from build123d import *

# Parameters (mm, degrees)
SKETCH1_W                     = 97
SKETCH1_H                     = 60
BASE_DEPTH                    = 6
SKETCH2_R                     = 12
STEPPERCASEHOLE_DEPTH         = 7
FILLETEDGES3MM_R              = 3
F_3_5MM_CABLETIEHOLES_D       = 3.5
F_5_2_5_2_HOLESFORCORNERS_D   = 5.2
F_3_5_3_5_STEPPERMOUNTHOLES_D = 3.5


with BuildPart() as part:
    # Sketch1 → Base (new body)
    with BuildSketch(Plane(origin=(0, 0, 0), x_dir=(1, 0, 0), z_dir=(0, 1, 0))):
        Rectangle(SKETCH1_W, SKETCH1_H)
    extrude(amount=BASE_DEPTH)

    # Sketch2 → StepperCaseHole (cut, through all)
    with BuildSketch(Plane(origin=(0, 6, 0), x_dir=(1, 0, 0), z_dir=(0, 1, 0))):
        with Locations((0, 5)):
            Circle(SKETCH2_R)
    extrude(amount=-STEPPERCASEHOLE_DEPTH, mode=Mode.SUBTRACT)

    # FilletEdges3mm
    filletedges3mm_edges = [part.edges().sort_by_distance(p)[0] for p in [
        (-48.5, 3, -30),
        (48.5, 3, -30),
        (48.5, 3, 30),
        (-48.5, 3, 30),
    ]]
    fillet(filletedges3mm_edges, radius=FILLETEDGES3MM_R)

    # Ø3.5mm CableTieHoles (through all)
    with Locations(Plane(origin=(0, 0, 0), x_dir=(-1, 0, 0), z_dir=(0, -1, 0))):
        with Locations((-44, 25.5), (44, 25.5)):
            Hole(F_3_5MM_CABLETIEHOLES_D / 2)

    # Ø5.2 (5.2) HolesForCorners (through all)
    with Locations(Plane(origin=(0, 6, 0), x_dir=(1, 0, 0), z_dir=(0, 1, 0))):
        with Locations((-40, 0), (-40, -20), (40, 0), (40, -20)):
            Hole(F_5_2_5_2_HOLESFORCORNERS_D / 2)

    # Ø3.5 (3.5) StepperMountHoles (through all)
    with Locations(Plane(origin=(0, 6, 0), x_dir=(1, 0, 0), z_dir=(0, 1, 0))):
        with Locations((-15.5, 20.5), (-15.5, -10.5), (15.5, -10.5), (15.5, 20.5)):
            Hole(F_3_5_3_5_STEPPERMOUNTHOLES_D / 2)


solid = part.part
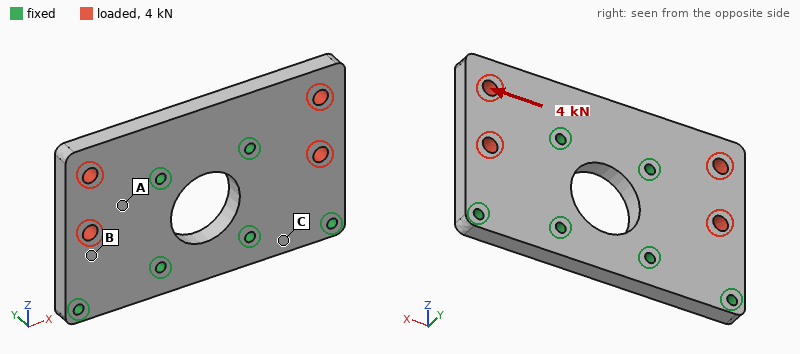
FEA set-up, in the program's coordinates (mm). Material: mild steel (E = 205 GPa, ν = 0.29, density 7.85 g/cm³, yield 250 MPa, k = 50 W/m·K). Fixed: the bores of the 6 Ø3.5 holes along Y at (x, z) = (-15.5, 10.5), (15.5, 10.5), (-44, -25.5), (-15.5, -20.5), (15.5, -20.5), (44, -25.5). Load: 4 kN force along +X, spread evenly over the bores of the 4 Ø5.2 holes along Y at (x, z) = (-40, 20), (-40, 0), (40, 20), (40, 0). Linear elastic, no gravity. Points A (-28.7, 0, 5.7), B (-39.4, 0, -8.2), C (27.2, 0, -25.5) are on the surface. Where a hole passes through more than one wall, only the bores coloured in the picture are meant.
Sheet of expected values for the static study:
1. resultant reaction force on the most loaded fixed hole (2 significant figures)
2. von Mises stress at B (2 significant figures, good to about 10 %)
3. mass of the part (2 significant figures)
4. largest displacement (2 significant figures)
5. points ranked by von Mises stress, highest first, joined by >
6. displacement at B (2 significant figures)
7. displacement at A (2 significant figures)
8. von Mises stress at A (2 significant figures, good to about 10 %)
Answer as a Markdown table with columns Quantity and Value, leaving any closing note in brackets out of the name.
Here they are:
| Quantity | Value |
|---|---|
| resultant reaction force on the most loaded fixed hole | 1.5 kN |
| von Mises stress at B | 5.1 MPa |
| mass of the part | 250 g |
| largest displacement | 2.2 µm |
| points ranked by von Mises stress, highest first, joined by > | A > B > C |
| displacement at B | 0.73 µm |
| displacement at A | 0.86 µm |
| von Mises stress at A | 9.9 MPa |
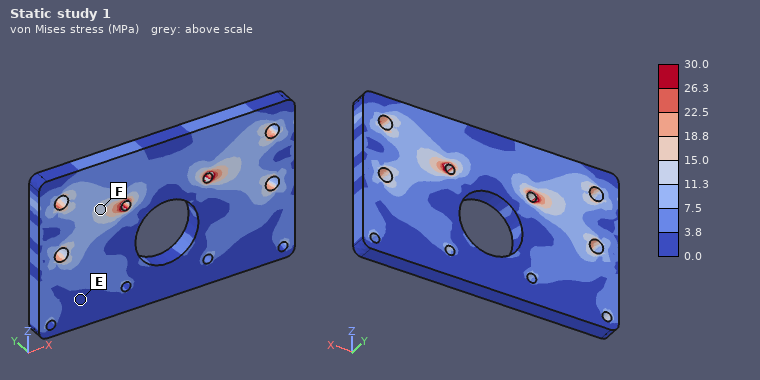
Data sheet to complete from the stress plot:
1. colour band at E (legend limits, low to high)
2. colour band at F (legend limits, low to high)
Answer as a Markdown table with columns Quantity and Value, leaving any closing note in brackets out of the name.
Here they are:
| Quantity | Value |
|---|---|
| colour band at E | 0.0 to 3.8 MPa |
| colour band at F | 11.3 to 15.0 MPa |
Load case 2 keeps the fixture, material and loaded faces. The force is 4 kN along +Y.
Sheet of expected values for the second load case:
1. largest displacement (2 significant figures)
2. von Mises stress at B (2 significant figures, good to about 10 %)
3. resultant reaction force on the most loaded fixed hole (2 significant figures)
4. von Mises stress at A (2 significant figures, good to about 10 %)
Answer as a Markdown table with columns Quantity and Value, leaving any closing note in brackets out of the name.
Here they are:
| Quantity | Value |
|---|---|
| largest displacement | 99 µm |
| von Mises stress at B | 76 MPa |
| resultant reaction force on the most loaded fixed hole | 1.5 kN |
| von Mises stress at A | 66 MPa |
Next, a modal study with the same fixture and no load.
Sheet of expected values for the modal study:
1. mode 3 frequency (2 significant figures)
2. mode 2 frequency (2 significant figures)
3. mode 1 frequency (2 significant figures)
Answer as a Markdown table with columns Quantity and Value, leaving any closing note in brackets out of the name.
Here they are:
| Quantity | Value |
|---|---|
| mode 3 frequency | 9700 Hz |
| mode 2 frequency | 5100 Hz |
| mode 1 frequency | 5000 Hz |
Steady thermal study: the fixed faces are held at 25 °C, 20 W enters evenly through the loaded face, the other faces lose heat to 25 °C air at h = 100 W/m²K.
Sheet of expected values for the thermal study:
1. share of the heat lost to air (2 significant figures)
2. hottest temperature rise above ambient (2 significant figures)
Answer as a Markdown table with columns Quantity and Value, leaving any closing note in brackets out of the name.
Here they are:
| Quantity | Value |
|---|---|
| share of the heat lost to air | 33 % |
| hottest temperature rise above ambient | 17 K |
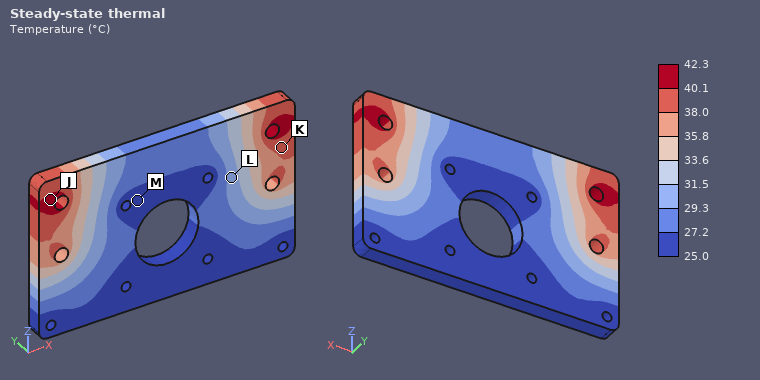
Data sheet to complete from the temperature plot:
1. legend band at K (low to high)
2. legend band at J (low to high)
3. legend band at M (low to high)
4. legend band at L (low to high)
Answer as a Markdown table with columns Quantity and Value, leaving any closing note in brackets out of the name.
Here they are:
| Quantity | Value |
|---|---|
| legend band at K | 38.0 to 40.1 °C |
| legend band at J | 40.1 to 42.3 °C |
| legend band at M | 25.0 to 27.2 °C |
| legend band at L | 29.3 to 31.5 °C |
